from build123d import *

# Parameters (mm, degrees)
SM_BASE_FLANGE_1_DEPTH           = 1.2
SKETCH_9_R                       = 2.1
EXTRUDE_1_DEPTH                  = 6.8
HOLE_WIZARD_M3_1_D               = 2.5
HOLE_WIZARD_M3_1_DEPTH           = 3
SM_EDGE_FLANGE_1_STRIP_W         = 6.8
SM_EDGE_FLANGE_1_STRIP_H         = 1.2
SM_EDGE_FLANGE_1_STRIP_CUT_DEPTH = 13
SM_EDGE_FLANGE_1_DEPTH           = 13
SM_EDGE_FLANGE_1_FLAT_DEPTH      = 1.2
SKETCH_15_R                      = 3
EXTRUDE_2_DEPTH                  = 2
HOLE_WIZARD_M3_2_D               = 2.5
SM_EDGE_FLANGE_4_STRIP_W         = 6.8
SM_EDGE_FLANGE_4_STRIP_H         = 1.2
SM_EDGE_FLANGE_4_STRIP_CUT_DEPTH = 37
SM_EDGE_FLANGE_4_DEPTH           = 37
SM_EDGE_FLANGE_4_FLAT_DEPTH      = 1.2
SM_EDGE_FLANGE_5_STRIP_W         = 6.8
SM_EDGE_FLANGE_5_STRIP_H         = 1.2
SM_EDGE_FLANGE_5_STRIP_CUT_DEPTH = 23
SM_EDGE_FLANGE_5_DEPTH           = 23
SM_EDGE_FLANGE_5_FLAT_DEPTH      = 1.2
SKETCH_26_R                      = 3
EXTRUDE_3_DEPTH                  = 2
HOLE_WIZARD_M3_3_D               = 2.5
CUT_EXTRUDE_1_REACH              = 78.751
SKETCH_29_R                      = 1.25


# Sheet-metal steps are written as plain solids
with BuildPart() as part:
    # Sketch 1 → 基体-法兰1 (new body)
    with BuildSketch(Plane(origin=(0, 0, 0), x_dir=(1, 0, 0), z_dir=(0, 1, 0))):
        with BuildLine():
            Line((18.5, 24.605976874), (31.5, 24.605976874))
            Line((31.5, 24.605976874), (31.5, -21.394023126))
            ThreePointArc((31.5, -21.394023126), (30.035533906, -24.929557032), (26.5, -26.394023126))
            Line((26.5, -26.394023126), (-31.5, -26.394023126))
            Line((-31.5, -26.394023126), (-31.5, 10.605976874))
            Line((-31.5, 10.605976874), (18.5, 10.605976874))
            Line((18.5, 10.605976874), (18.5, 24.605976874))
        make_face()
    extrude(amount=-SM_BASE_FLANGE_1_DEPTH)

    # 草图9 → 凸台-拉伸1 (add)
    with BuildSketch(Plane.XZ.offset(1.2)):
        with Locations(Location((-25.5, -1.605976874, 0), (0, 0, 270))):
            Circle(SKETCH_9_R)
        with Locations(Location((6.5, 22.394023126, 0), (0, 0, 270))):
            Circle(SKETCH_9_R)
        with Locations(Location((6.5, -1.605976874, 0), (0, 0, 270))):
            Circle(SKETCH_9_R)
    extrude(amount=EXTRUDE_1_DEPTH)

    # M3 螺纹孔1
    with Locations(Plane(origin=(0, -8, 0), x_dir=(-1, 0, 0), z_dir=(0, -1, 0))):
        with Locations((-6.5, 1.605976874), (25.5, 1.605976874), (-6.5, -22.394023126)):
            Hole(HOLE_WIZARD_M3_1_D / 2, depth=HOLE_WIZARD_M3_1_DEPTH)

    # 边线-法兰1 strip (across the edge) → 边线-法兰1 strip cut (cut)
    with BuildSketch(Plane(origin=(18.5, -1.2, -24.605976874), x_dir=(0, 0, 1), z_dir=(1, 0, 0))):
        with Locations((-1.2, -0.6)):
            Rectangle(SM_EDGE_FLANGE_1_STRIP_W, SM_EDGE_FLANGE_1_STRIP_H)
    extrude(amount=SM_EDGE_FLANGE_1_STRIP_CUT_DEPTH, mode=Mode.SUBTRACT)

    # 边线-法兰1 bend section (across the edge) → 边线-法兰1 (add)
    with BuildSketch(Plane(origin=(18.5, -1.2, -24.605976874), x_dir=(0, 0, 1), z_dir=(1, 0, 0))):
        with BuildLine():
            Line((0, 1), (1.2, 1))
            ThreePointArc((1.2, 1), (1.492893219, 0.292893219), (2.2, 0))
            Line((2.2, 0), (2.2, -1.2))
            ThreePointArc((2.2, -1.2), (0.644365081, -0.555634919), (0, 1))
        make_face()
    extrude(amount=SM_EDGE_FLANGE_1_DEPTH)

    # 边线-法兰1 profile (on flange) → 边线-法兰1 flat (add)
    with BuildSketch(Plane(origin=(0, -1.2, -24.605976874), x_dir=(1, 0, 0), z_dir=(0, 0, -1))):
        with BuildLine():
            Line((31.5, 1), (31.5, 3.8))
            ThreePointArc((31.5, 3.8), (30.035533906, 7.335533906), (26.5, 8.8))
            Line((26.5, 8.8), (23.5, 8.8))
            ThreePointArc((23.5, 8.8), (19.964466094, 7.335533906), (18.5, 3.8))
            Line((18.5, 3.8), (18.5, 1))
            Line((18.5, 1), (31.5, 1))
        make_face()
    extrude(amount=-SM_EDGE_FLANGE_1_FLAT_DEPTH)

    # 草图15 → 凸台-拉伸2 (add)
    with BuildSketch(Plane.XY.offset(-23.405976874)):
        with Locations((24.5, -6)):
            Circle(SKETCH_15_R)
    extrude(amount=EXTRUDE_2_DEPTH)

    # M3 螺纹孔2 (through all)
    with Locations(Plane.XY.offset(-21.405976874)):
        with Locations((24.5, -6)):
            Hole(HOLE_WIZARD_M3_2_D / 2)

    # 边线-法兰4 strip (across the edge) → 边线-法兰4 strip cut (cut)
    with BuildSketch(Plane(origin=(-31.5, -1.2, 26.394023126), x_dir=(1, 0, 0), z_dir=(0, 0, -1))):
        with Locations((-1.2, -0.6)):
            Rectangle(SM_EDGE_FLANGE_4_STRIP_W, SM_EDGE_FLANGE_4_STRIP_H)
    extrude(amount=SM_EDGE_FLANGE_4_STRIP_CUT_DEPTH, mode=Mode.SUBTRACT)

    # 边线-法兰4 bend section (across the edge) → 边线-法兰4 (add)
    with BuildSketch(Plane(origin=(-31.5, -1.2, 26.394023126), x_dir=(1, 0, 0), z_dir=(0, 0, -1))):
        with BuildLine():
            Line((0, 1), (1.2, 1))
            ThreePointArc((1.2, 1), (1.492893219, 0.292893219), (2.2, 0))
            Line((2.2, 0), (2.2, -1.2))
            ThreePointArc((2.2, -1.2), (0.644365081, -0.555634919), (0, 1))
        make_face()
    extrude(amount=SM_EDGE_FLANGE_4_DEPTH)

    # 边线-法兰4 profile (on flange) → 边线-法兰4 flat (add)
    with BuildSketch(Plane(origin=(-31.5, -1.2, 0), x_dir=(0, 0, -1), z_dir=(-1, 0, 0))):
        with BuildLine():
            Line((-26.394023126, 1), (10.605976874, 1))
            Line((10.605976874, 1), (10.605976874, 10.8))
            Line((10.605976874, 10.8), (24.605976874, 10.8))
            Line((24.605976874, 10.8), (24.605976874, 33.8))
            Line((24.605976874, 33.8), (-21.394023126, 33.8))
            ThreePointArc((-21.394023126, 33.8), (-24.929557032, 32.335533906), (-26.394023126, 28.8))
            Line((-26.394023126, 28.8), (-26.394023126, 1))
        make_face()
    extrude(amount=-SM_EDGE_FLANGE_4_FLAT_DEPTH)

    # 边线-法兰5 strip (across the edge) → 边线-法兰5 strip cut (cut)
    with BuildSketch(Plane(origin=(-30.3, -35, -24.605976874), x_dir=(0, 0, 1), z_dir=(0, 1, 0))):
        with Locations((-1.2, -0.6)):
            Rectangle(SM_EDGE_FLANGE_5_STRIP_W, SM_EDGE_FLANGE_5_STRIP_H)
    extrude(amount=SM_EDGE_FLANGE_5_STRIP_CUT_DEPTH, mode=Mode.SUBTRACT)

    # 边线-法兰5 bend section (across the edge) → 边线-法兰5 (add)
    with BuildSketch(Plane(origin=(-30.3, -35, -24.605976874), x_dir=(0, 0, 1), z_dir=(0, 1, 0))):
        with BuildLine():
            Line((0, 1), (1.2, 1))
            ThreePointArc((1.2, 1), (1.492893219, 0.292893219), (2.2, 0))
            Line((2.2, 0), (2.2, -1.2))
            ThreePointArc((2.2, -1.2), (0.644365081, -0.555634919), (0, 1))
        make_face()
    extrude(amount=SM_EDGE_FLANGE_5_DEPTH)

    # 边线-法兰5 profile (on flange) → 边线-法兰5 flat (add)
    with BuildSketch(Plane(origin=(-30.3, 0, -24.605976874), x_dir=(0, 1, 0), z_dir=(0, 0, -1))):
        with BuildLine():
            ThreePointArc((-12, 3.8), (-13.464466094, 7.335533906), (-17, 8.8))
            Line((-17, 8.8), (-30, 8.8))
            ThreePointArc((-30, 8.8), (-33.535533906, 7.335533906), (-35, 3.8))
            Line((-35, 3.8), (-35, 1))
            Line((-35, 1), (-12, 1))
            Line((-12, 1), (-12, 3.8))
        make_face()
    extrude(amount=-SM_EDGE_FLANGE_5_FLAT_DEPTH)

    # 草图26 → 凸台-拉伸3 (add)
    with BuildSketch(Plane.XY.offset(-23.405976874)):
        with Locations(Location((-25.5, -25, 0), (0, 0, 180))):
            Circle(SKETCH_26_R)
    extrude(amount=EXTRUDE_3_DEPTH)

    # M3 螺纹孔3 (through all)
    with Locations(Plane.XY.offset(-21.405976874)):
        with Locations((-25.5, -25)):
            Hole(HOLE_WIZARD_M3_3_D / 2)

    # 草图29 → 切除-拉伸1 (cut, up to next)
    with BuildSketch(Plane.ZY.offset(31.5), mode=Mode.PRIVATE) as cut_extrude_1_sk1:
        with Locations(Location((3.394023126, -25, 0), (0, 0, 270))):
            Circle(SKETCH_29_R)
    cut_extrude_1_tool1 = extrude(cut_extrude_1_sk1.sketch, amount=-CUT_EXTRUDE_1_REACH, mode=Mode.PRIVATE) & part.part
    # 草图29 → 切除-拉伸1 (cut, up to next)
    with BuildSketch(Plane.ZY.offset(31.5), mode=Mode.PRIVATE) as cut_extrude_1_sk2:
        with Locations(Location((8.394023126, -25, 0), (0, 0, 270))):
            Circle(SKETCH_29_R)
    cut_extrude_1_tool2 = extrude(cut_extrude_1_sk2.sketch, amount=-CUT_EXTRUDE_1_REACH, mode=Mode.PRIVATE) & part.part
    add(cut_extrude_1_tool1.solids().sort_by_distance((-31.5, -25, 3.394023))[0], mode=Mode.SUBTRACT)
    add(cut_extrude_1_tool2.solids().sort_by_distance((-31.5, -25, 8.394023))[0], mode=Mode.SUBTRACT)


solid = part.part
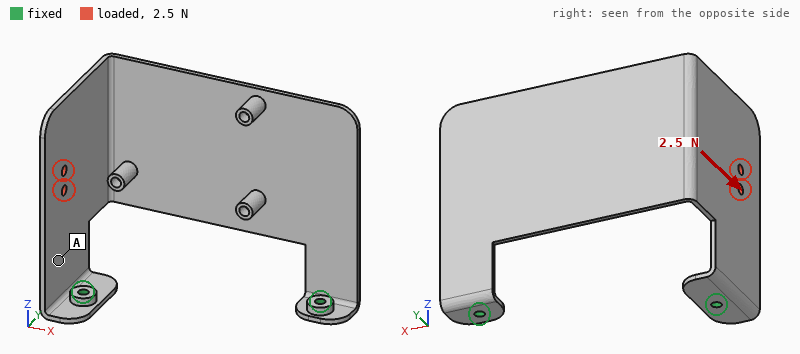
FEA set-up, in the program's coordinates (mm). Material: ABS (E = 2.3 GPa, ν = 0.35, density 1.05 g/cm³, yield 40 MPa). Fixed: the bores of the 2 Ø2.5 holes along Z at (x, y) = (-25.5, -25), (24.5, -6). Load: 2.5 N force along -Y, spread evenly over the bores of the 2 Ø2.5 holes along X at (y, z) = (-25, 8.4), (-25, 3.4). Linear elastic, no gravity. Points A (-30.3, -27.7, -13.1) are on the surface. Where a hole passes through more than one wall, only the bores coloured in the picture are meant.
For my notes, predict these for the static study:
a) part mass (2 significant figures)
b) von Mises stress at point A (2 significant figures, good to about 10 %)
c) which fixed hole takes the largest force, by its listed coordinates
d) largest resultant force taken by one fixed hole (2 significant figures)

5.8 g
0.72 MPa
(-25.5, -25)
2.5 N
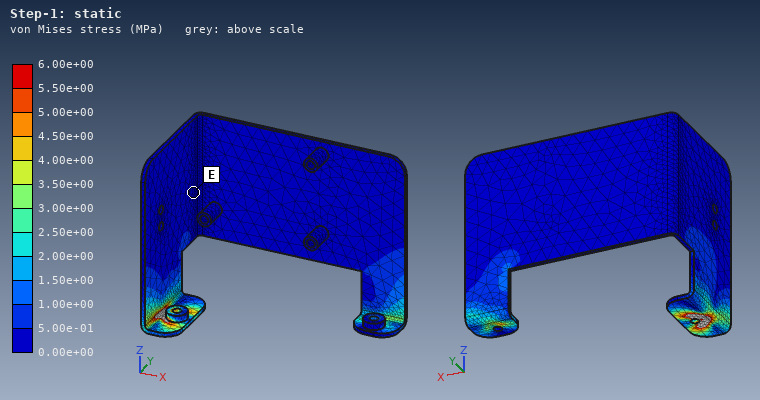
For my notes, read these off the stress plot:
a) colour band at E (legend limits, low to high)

0.00e+00 to 5.00e-01 MPa
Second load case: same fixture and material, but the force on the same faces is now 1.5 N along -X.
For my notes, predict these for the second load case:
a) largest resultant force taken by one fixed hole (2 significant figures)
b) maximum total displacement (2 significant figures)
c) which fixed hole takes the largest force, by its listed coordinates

0.97 N
1.0 mm
(-25.5, -25)
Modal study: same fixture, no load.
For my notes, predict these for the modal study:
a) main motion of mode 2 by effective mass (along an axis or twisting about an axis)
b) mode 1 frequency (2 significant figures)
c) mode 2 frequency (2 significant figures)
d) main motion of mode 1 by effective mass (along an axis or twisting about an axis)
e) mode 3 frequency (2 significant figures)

along X
110 Hz
180 Hz
along Y
270 Hz
